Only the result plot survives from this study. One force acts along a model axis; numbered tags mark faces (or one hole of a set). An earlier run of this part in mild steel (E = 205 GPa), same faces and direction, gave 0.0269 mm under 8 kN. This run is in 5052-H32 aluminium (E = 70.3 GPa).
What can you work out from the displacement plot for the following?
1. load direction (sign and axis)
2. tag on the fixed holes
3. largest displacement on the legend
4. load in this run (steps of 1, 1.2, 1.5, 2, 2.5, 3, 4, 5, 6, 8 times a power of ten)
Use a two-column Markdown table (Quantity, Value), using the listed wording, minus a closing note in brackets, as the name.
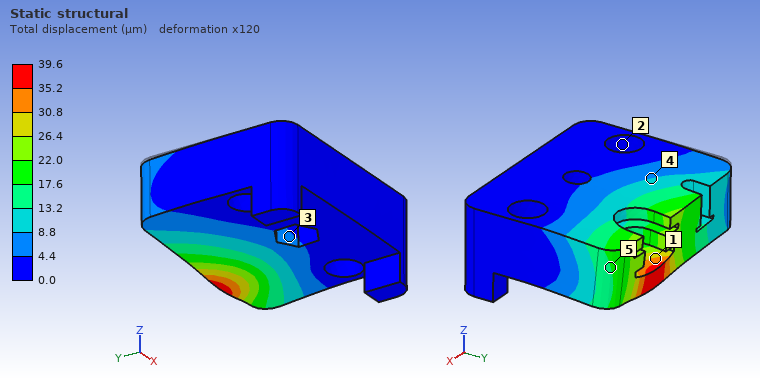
| Quantity | Value |
|---|---|
| load direction | -Z |
| tag on the fixed holes | 2 |
| largest displacement on the legend | 39.6 µm |
| load in this run | 4 kN |
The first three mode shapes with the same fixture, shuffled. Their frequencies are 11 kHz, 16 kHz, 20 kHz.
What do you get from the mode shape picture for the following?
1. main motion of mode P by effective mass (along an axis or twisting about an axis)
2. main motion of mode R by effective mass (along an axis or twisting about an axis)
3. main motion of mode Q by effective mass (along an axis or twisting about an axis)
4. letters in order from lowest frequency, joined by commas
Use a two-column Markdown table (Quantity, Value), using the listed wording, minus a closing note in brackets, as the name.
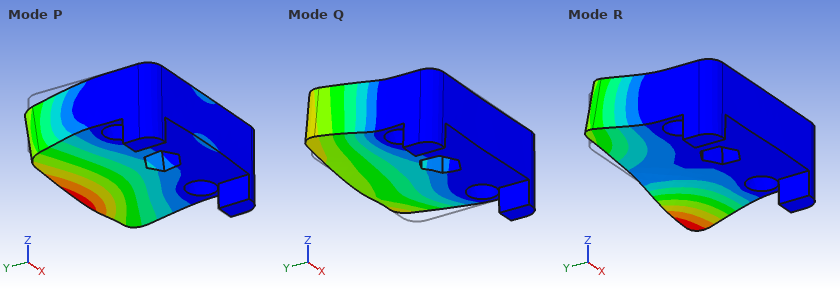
| Quantity | Value |
|---|---|
| main motion of mode P by effective mass | along Z |
| main motion of mode R by effective mass | twisting about Y |
| main motion of mode Q by effective mass | along X |
| letters in order from lowest frequency, joined by commas | P, R, Q |
